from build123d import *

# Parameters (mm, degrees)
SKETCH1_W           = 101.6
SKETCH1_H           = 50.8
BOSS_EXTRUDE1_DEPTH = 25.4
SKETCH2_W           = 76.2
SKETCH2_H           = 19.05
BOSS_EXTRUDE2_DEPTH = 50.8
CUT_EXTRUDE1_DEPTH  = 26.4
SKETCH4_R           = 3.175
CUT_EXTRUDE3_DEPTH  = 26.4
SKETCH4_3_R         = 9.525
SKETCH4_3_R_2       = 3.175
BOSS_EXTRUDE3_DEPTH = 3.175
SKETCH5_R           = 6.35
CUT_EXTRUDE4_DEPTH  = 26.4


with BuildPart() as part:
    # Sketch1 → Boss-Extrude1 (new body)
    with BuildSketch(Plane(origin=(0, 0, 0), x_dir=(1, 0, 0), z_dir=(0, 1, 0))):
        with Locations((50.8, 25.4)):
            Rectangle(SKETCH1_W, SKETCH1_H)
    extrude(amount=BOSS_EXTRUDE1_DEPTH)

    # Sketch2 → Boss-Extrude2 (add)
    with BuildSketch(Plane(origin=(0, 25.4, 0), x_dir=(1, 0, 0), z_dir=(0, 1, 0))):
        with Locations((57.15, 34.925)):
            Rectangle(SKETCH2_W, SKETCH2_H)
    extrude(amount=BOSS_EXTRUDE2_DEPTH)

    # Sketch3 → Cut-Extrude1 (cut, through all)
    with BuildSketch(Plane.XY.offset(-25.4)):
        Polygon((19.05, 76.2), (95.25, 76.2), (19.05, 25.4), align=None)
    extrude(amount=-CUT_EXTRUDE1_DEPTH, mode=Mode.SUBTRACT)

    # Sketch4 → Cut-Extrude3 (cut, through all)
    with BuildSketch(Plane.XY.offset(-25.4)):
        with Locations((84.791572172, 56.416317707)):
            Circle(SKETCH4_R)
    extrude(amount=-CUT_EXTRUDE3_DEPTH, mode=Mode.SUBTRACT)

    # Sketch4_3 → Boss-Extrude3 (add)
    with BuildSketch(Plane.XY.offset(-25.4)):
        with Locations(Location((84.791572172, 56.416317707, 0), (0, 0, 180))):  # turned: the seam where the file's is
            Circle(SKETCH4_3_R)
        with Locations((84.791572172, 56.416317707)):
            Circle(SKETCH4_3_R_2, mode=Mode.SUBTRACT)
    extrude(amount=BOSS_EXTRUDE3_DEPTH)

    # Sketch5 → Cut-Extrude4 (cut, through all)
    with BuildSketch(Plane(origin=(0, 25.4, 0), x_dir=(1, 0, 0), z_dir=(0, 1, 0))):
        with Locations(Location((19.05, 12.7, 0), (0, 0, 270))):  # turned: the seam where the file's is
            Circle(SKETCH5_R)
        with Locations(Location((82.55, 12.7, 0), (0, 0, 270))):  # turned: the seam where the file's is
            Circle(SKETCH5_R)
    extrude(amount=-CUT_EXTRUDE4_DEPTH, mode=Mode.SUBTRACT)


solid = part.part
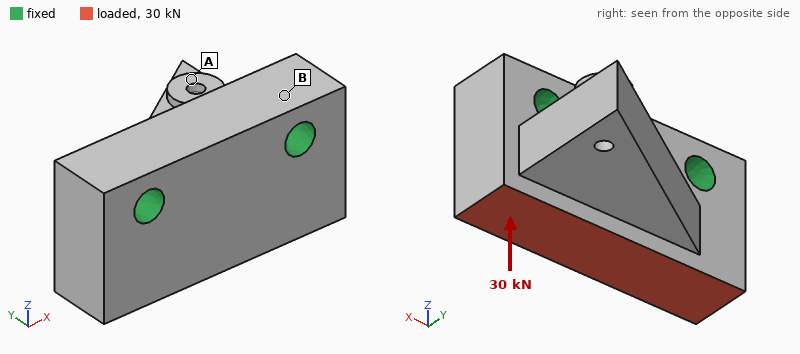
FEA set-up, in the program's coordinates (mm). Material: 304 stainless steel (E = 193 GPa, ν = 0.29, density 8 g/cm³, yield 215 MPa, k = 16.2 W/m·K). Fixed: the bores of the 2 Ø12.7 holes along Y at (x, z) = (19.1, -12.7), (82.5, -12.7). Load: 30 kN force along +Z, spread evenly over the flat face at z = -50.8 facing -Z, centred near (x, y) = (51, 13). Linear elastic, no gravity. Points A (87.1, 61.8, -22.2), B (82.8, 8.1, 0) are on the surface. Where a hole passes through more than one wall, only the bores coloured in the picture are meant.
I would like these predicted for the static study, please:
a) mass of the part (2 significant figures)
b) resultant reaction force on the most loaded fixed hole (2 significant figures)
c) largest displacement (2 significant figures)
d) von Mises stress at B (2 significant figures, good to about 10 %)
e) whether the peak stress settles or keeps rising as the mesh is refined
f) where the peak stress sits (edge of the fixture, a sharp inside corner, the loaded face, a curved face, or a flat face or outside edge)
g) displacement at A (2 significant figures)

1.3 kg
15 kN
3.5 µm
11 MPa
keeps rising
edge of the fixture
1.5 µm
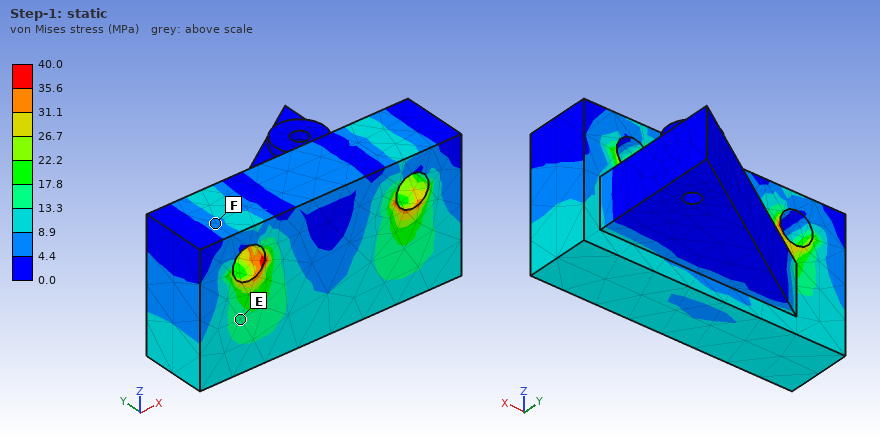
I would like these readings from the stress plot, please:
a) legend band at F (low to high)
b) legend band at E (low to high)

4.4 to 8.9 MPa
13.3 to 17.8 MPa
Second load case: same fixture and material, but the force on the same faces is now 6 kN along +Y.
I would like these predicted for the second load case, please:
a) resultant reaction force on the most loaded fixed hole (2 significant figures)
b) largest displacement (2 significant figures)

3.0 kN
12 µm
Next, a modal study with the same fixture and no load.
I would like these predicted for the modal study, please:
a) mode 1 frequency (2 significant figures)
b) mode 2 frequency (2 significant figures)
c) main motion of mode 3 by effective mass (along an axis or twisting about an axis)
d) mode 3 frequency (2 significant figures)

5200 Hz
9300 Hz
along Y
10 kHz
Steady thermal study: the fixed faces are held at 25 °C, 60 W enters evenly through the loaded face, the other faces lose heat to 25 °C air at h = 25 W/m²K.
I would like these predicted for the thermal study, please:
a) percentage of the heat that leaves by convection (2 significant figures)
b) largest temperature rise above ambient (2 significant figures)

17 %
51 K
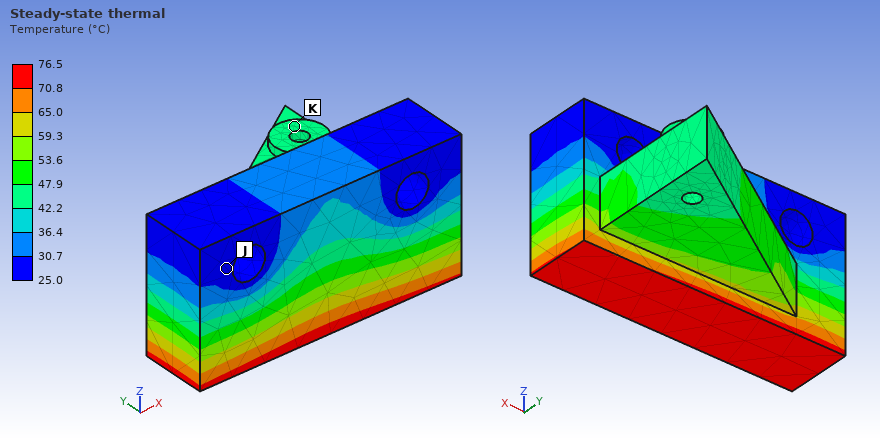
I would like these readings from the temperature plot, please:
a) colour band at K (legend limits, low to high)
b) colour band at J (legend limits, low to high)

42.2 to 47.9 °C
25.0 to 30.7 °C
